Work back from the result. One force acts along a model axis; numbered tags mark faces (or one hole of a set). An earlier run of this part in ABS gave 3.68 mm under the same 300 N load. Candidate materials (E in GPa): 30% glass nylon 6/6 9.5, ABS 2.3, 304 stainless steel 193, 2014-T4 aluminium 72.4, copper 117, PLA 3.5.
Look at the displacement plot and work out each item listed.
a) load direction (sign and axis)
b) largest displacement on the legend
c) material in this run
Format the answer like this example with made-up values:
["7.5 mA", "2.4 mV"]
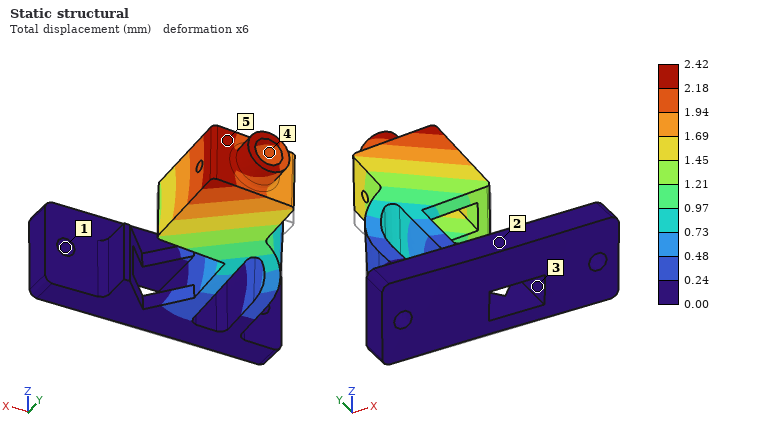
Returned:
["+Z", "2.42 mm", "PLA"]
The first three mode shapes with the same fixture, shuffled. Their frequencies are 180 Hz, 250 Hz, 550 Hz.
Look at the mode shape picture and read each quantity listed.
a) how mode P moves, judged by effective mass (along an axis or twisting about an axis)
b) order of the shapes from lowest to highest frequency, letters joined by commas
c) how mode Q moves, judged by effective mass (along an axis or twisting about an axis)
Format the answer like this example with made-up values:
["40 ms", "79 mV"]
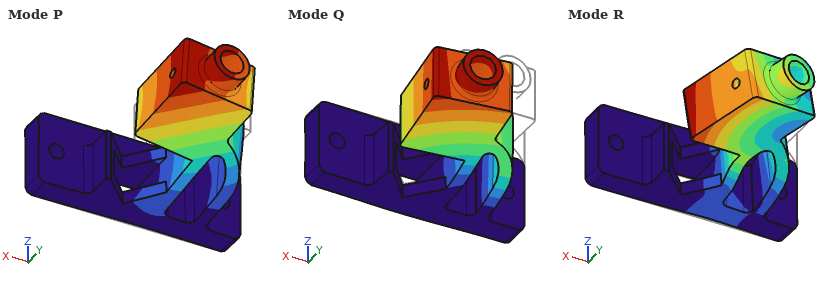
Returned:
["along Z", "P, Q, R", "along X"]
